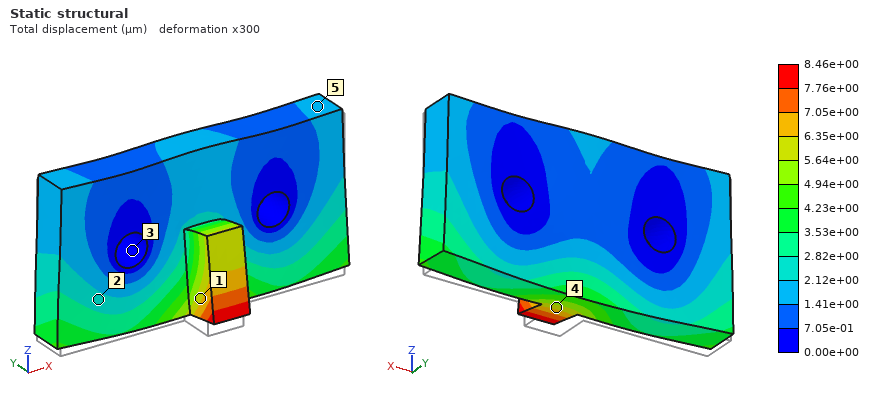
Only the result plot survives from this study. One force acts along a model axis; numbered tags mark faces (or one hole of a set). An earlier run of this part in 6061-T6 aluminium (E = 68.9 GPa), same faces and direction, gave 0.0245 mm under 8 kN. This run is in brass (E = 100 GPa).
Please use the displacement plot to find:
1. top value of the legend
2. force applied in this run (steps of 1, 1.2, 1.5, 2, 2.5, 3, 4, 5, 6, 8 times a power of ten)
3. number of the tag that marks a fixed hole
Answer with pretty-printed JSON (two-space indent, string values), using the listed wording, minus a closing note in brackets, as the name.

{
  "top value of the legend": "8.46e+00 µm",
  "force applied in this run": "4 kN",
  "number of the tag that marks a fixed hole": "3"
}
